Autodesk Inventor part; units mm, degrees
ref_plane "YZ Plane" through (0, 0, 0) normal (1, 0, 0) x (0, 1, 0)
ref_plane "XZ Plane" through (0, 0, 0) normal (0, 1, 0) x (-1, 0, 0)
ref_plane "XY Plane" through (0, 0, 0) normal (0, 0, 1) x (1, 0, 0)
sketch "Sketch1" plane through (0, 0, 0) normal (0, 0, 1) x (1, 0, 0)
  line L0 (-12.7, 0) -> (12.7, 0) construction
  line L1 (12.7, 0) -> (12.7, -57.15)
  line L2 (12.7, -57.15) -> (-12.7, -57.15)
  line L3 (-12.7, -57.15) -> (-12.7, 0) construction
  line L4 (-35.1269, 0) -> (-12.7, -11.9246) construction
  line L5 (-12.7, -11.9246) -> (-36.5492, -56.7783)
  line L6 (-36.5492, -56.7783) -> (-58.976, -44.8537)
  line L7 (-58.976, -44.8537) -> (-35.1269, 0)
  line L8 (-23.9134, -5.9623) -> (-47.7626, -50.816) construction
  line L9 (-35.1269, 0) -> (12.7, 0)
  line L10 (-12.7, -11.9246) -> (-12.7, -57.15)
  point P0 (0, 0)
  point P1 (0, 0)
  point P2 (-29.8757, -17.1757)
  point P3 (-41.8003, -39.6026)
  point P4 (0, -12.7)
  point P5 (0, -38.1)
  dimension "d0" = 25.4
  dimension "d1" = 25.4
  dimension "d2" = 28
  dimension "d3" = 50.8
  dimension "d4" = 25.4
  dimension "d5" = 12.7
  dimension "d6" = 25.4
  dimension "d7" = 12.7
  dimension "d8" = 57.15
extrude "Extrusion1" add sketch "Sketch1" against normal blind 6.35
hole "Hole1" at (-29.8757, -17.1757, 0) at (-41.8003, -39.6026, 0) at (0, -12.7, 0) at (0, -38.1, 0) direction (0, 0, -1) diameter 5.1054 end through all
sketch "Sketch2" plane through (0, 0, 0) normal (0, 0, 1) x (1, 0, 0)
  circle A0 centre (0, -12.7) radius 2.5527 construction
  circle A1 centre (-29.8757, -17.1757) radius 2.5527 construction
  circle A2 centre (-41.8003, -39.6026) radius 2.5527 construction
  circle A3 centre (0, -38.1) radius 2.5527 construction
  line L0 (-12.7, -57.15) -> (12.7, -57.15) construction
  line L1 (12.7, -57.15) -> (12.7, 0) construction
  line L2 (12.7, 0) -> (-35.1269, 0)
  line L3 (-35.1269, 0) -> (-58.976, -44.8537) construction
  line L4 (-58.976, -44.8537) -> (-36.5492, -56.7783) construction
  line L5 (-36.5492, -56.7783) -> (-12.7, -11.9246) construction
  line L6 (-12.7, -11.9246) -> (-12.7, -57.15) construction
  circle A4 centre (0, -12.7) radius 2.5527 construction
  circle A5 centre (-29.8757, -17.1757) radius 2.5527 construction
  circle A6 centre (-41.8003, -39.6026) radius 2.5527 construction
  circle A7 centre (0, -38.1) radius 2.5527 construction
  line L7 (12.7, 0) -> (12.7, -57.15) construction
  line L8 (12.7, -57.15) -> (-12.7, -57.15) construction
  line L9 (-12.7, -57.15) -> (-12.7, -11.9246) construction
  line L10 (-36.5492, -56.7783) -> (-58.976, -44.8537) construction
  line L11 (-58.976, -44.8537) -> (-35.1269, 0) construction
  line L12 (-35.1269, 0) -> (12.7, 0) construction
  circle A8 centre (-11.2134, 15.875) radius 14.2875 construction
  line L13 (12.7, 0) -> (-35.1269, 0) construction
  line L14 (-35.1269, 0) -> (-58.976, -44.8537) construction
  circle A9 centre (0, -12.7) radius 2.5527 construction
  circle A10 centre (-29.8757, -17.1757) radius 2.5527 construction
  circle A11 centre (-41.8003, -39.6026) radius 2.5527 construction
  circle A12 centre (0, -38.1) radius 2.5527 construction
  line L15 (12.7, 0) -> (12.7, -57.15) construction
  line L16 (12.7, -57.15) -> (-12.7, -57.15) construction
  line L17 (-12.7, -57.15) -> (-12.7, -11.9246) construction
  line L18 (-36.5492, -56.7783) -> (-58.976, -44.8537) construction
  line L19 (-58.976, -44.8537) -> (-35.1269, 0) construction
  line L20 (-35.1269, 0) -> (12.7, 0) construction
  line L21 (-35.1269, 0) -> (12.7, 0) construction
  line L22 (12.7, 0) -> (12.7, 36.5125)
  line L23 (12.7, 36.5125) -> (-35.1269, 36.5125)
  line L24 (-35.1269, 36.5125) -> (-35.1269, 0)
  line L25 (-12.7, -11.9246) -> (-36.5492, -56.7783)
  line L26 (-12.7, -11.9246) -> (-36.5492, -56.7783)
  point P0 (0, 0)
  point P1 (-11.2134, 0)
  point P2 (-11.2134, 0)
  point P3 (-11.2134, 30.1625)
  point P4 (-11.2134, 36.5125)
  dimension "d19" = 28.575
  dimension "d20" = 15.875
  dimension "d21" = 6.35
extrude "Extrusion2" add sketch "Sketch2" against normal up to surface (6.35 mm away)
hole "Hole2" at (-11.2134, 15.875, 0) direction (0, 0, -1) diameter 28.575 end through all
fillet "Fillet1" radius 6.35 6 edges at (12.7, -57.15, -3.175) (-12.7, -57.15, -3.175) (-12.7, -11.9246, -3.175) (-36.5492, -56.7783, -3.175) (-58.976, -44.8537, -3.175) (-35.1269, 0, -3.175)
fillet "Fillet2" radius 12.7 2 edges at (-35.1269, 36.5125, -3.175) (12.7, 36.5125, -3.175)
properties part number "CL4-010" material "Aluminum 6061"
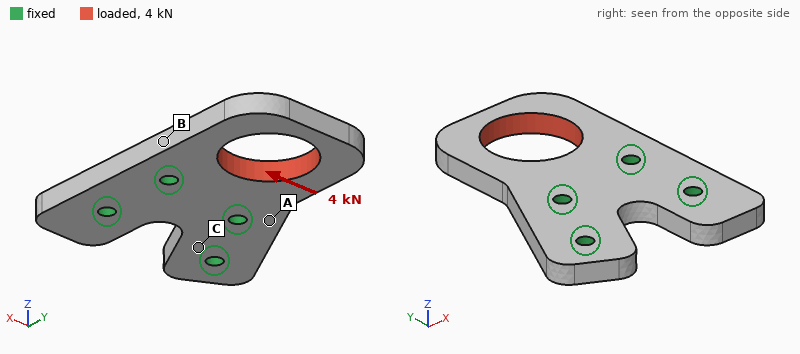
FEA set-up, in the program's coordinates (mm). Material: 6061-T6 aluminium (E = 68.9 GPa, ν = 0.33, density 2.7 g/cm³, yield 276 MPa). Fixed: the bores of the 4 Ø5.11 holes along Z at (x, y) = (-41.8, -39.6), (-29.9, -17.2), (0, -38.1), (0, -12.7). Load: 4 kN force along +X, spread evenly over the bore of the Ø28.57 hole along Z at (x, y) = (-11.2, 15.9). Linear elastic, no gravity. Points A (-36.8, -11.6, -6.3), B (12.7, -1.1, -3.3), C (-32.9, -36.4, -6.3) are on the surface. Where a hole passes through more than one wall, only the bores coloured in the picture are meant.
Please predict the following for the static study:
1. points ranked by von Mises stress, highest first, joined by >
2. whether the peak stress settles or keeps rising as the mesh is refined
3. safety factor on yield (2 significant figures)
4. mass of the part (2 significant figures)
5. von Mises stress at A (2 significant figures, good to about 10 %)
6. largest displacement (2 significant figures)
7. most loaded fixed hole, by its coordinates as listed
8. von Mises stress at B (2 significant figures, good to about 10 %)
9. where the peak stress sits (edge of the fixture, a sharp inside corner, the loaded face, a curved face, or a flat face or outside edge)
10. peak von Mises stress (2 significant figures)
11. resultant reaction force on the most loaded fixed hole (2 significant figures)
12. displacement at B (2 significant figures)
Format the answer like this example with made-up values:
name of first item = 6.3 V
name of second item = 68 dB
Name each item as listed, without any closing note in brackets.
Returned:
points ranked by von Mises stress, highest first, joined by > = B > A > C
whether the peak stress settles or keeps rising as the mesh is refined = settles
safety factor on yield = 2.5
mass of the part = 67 g
von Mises stress at A = 28 MPa
largest displacement = 0.11 mm
most loaded fixed hole, by its coordinates as listed = (0, -12.7)
von Mises stress at B = 67 MPa
where the peak stress sits = the loaded face
peak von Mises stress = 110 MPa
resultant reaction force on the most loaded fixed hole = 3.5 kN
displacement at B = 0.024 mm
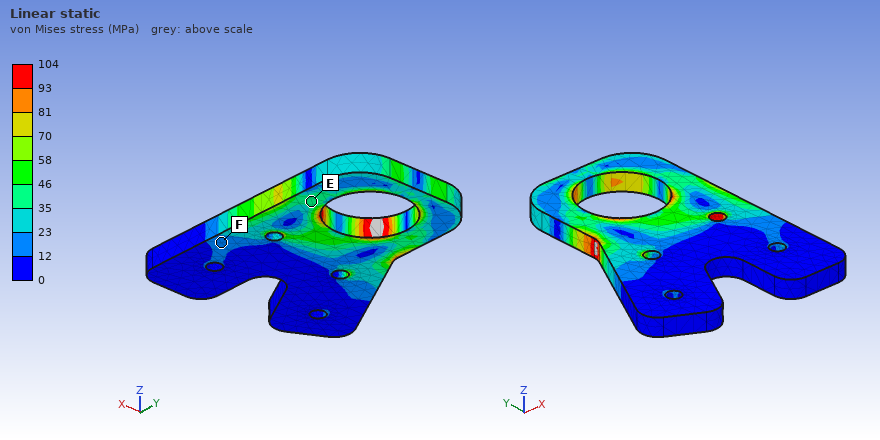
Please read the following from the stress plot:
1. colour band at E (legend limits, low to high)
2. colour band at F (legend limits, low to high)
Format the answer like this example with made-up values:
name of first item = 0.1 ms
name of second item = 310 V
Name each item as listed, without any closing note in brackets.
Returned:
colour band at E = 35 to 46 MPa
colour band at F = 12 to 23 MPa
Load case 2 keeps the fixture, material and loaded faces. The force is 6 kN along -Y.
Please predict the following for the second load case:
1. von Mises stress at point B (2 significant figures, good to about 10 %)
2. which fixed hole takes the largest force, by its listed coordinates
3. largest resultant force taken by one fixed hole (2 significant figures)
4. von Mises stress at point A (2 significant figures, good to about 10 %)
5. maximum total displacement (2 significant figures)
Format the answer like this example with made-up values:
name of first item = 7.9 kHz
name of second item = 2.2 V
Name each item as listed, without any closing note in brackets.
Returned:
von Mises stress at point B = 36 MPa
which fixed hole takes the largest force, by its listed coordinates = (0, -12.7)
largest resultant force taken by one fixed hole = 2.9 kN
von Mises stress at point A = 14 MPa
maximum total displacement = 42 µm
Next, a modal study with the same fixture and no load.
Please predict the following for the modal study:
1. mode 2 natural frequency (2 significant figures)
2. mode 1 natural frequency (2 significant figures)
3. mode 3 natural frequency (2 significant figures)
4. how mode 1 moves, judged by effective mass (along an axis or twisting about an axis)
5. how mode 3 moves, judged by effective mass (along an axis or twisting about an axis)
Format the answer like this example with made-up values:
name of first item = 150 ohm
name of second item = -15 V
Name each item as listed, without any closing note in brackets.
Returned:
mode 2 natural frequency = 4500 Hz
mode 1 natural frequency = 2200 Hz
mode 3 natural frequency = 7500 Hz
how mode 1 moves, judged by effective mass = along Z
how mode 3 moves, judged by effective mass = along X
